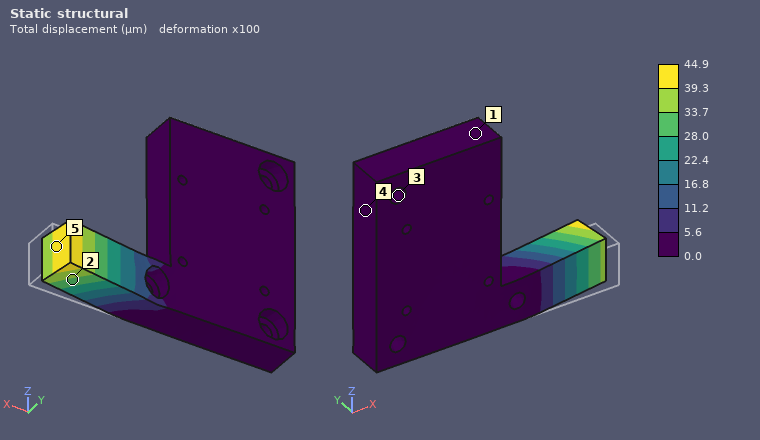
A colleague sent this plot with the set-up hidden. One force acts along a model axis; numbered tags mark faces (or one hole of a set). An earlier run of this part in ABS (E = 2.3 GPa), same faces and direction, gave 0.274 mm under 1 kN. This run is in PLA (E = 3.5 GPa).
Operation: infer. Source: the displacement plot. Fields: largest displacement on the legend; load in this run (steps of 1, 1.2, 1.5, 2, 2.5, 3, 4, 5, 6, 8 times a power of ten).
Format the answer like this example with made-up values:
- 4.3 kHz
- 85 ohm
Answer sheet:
- 44.9 µm
- 250 N
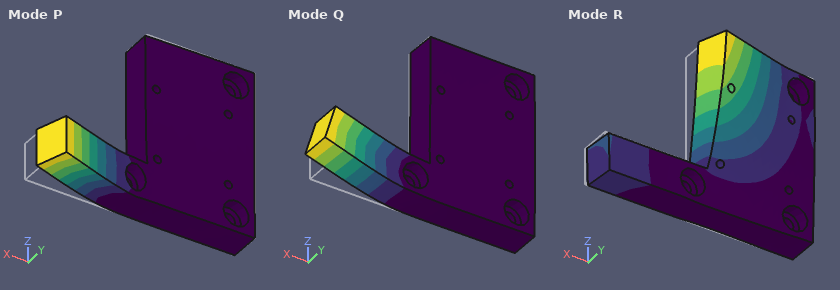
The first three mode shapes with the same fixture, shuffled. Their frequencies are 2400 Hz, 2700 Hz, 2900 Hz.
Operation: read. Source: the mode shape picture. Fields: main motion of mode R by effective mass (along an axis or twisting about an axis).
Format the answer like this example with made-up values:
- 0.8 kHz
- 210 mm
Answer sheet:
- along Y
